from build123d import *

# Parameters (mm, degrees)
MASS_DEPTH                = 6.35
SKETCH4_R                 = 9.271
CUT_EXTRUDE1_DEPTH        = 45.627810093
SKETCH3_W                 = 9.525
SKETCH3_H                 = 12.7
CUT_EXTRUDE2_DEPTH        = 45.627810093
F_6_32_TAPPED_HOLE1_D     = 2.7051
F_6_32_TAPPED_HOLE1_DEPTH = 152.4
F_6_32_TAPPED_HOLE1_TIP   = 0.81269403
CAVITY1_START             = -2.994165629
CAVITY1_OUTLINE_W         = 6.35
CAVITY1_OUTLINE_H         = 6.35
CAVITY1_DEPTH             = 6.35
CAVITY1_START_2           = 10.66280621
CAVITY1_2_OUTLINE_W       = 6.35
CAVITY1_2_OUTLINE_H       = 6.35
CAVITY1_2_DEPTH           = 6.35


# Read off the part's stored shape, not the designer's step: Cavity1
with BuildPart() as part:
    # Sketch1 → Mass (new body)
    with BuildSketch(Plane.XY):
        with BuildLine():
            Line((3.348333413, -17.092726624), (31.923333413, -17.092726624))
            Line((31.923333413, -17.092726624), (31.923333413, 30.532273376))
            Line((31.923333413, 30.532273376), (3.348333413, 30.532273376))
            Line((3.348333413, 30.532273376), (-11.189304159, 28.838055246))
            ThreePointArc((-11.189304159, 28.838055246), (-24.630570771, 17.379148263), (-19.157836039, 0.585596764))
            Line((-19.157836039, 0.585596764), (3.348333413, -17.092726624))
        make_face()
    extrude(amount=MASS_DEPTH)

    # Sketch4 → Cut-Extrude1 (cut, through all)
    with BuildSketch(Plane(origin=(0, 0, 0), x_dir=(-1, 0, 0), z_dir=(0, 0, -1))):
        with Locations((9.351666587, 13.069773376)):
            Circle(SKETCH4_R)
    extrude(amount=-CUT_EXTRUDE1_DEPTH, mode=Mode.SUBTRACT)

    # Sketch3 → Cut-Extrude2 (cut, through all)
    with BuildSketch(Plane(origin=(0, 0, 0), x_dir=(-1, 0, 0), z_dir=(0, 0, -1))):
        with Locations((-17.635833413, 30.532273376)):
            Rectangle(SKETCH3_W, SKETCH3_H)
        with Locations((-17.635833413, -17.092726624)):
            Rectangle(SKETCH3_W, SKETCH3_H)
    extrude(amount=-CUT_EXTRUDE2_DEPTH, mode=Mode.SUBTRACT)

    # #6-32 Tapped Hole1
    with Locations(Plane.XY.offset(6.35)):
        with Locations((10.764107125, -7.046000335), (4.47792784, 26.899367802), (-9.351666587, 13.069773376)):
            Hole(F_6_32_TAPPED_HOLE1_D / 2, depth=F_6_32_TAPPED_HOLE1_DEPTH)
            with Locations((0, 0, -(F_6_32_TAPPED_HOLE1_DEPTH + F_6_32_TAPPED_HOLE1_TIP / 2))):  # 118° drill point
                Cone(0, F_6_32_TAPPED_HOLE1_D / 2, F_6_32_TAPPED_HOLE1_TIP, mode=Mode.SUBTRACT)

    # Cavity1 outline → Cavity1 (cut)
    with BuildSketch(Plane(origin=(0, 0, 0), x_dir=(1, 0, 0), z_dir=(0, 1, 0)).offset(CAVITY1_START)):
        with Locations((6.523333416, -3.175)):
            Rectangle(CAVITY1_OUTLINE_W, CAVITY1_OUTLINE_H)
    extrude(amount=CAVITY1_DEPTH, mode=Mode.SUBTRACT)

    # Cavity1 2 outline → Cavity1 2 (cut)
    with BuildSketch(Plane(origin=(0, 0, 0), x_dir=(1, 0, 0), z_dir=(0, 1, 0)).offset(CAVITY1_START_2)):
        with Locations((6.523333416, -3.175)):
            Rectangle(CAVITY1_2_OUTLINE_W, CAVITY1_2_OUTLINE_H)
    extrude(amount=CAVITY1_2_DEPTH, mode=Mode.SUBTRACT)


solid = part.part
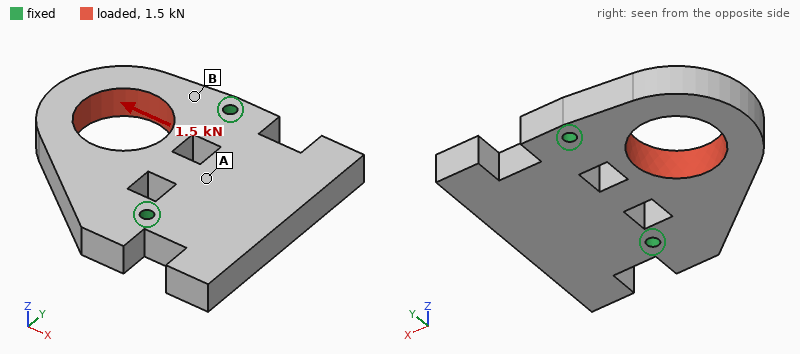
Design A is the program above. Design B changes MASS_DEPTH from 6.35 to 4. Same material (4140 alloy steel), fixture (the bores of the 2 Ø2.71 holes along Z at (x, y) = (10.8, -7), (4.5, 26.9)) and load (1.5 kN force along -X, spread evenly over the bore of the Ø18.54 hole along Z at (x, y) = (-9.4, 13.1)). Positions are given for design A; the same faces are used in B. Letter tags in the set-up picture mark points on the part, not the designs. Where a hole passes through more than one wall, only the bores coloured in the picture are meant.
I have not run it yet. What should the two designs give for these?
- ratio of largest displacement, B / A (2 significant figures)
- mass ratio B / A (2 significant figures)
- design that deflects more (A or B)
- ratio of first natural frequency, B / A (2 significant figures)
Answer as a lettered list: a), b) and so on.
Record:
a) 1.6
b) 0.63
c) B
d) 0.68
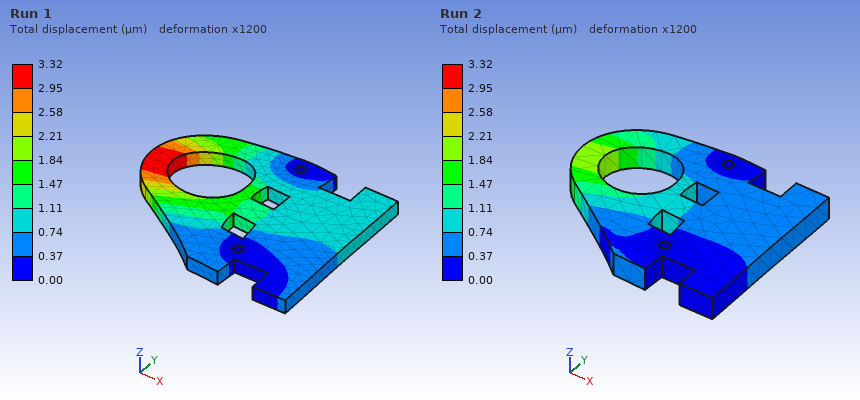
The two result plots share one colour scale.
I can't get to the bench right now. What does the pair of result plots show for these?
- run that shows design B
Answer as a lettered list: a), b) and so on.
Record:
a) Run 1
